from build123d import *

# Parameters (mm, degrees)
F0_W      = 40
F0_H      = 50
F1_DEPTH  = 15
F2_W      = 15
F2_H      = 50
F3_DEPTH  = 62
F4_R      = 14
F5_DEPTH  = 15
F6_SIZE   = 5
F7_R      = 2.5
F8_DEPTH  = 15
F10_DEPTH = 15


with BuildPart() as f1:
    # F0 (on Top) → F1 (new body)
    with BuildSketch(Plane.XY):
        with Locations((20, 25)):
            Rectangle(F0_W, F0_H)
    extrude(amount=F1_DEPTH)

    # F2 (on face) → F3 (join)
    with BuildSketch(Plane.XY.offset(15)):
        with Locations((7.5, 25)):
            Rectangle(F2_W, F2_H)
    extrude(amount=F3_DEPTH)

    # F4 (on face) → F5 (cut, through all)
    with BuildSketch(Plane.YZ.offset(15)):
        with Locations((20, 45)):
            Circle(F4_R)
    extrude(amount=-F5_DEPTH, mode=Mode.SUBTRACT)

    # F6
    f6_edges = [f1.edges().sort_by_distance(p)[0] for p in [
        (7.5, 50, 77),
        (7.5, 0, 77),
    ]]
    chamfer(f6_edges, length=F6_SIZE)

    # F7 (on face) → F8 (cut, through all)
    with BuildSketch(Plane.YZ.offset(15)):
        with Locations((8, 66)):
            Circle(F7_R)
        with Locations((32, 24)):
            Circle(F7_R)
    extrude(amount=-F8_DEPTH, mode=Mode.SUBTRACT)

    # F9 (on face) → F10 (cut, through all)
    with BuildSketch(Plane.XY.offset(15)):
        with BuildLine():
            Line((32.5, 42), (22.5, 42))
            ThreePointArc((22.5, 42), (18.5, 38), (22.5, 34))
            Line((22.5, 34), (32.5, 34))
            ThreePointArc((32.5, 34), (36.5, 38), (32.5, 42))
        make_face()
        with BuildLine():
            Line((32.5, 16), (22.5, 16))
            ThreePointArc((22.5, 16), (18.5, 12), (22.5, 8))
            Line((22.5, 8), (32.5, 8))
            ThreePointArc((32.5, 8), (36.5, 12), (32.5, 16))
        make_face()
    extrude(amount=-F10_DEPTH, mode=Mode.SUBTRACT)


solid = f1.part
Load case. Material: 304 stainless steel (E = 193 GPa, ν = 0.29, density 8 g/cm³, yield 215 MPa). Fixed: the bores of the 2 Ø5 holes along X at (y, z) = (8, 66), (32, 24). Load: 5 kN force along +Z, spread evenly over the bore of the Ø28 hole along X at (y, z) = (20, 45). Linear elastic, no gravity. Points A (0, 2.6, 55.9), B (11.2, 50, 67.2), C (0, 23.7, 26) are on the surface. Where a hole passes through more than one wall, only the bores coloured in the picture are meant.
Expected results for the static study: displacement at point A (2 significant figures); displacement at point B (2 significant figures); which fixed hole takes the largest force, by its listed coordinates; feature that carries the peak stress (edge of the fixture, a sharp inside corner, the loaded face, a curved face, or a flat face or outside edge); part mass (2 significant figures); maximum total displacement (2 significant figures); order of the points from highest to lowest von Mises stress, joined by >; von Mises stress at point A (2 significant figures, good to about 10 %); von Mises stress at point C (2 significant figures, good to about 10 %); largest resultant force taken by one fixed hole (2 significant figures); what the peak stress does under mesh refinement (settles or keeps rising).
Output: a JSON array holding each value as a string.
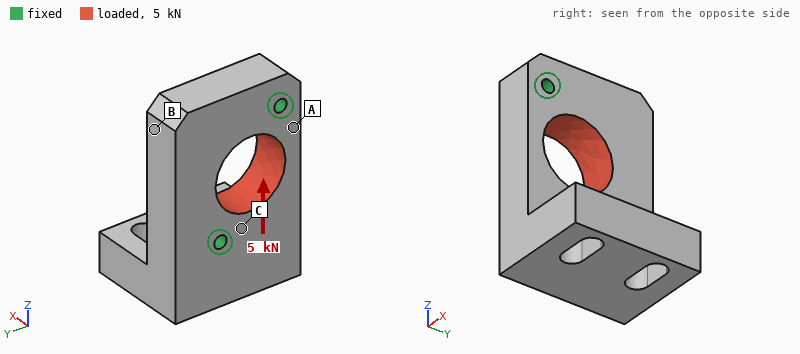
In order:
["0.52 µm", "0.80 µm", "(32, 24)", "edge of the fixture", "500 g", "1.6 µm", "A > C > B", "9.1 MPa", "4.6 MPa", "2.7 kN", "keeps rising"]
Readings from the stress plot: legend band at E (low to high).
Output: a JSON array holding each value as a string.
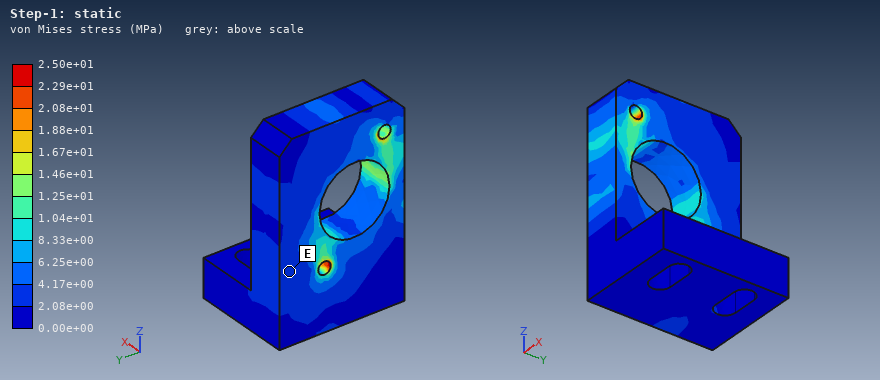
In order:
["2.08e+00 to 4.17e+00 MPa"]
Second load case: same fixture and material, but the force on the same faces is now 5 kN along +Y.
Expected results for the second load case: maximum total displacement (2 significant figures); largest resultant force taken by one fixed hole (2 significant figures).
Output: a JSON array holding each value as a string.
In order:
["2.4 µm", "2.5 kN"]
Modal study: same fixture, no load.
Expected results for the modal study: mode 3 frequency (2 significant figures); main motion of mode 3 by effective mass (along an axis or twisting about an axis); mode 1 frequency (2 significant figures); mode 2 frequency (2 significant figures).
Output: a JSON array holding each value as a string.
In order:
["7600 Hz", "along X", "4600 Hz", "5900 Hz"]
